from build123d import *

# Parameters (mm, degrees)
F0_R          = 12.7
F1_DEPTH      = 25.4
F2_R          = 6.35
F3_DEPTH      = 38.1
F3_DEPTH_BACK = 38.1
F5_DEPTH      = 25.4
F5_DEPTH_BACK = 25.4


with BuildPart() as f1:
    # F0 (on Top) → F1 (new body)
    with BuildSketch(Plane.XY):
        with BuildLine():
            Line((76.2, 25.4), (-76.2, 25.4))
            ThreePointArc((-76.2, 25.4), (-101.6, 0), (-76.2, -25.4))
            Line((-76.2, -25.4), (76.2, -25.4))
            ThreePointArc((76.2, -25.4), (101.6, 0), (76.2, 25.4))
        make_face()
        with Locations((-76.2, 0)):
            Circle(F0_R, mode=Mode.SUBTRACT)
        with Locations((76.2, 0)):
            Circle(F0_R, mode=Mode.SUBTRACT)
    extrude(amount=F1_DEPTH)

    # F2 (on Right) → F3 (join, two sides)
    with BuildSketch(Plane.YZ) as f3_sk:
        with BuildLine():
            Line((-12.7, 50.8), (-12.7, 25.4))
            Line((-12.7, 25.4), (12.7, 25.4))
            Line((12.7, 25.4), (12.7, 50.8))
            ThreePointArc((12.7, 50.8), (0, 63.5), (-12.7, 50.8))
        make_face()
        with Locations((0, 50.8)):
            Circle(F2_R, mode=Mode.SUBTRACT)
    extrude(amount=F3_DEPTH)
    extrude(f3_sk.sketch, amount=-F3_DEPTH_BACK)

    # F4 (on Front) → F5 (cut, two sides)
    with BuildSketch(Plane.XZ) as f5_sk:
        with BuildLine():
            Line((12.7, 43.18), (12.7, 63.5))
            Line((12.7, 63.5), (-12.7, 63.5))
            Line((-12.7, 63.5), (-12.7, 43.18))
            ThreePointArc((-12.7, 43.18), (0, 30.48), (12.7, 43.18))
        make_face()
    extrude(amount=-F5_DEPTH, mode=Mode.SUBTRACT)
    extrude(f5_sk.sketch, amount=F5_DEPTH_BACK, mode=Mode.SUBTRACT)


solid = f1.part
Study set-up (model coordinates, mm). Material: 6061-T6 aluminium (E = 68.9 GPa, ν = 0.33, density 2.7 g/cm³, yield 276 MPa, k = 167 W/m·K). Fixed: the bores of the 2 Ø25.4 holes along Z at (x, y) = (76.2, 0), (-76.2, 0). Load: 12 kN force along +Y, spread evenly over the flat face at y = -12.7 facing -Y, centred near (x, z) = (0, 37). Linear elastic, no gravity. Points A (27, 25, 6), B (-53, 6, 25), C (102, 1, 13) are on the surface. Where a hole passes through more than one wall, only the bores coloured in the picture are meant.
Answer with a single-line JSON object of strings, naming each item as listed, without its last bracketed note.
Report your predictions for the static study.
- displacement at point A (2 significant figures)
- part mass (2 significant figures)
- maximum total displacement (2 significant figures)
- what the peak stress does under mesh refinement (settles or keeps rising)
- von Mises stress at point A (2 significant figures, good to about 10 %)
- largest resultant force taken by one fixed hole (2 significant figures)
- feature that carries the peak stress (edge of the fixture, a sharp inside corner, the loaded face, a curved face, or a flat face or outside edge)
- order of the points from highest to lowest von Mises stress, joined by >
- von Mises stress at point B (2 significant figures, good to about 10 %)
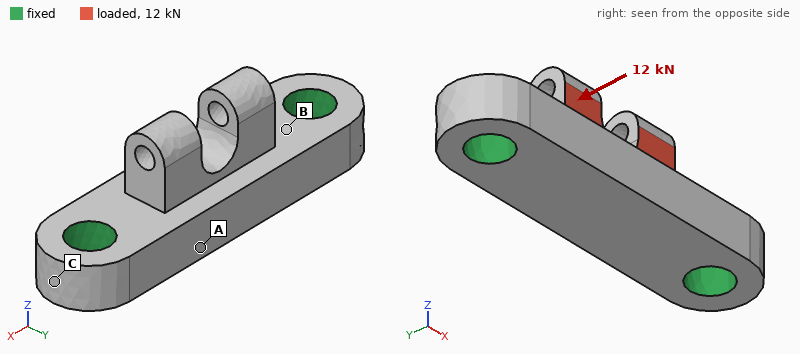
{"displacement at point A": "25 µm", "part mass": "720 g", "maximum total displacement": "85 µm", "what the peak stress does under mesh refinement": "keeps rising", "von Mises stress at point A": "14 MPa", "largest resultant force taken by one fixed hole": "6.0 kN", "feature that carries the peak stress": "edge of the fixture", "order of the points from highest to lowest von Mises stress, joined by >": "B > A > C", "von Mises stress at point B": "34 MPa"}
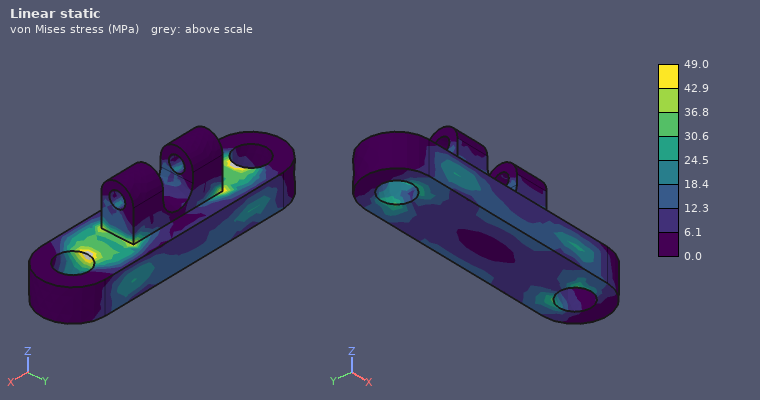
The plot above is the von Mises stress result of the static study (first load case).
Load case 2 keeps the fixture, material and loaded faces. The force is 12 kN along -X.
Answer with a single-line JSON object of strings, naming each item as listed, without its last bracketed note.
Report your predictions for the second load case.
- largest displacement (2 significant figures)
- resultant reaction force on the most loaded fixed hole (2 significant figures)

{"largest displacement": "27 µm", "resultant reaction force on the most loaded fixed hole": "6.7 kN"}
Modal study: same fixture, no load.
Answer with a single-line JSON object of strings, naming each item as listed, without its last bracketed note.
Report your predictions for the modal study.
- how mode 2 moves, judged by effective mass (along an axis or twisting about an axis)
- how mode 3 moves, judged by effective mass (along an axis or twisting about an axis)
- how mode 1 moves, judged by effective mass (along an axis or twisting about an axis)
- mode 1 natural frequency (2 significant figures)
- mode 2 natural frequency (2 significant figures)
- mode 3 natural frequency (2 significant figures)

{"how mode 2 moves, judged by effective mass": "along Z", "how mode 3 moves, judged by effective mass": "along Y", "how mode 1 moves, judged by effective mass": "along Y", "mode 1 natural frequency": "5200 Hz", "mode 2 natural frequency": "5400 Hz", "mode 3 natural frequency": "7700 Hz"}
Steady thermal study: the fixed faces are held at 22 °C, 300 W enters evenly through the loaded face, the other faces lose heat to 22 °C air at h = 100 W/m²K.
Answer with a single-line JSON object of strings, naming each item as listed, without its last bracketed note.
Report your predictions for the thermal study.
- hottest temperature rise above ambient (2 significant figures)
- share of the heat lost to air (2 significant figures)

{"hottest temperature rise above ambient": "49 K", "share of the heat lost to air": "20 %"}
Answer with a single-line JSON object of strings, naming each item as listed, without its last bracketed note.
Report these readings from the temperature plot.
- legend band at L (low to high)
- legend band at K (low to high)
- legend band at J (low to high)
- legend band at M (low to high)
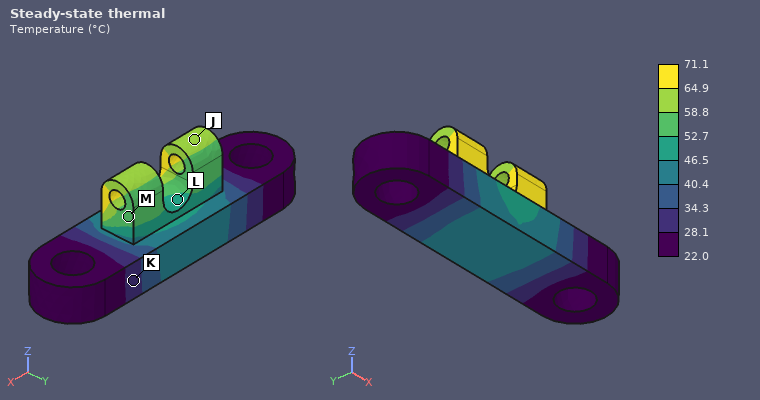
{"legend band at L": "46.5 to 52.7 °C", "legend band at K": "28.1 to 34.3 °C", "legend band at J": "58.8 to 64.9 °C", "legend band at M": "52.7 to 58.8 °C"}
